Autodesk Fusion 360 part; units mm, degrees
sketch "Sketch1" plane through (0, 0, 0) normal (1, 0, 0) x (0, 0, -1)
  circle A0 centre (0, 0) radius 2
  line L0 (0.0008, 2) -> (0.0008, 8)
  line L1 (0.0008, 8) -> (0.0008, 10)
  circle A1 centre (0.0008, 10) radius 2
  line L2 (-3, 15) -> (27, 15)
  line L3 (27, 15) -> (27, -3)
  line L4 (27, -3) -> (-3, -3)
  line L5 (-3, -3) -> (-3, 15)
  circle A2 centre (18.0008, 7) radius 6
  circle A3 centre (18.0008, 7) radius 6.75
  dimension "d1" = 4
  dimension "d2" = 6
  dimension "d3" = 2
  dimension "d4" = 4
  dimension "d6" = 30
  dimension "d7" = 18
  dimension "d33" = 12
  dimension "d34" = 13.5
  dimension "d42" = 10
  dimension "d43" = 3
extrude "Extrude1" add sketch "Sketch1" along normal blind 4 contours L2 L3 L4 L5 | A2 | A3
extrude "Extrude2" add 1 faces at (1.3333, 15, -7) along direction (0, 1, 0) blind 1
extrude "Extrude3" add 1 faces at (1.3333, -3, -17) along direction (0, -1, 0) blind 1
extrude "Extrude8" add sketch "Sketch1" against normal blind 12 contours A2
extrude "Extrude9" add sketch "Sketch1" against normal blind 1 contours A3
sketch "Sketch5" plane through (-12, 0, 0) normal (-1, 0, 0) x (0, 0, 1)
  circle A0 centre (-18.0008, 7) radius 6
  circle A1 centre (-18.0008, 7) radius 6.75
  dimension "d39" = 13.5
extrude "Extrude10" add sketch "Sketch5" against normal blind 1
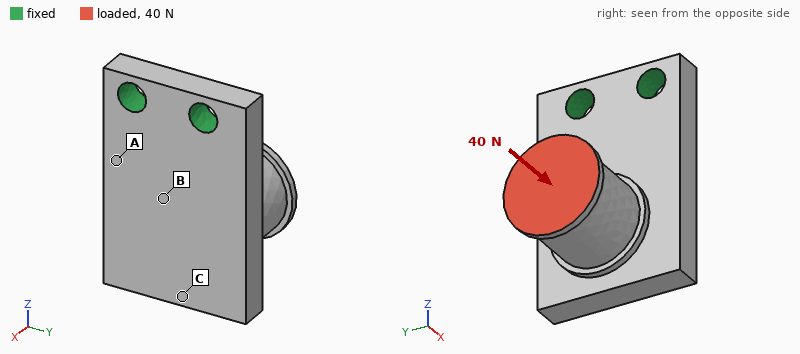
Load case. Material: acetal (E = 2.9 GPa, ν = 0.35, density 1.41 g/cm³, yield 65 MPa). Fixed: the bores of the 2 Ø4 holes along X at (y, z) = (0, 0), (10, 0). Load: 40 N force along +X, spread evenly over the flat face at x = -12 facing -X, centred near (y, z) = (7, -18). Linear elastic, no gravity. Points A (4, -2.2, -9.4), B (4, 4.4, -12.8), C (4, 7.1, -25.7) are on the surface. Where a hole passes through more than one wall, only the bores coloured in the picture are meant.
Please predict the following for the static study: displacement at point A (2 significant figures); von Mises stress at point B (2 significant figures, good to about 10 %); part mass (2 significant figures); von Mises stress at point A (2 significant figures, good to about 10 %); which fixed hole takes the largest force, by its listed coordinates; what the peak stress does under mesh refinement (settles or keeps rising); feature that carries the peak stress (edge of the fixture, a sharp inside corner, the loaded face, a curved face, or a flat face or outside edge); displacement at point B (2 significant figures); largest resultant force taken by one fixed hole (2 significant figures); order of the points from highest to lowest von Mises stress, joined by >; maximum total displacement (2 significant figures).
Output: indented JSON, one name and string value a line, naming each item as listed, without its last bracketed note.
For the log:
{
  "displacement at point A": "0.064 mm",
  "von Mises stress at point B": "3.6 MPa",
  "part mass": "5.2 g",
  "von Mises stress at point A": "6.4 MPa",
  "which fixed hole takes the largest force, by its listed coordinates": "(10, 0)",
  "what the peak stress does under mesh refinement": "keeps rising",
  "feature that carries the peak stress": "edge of the fixture",
  "displacement at point B": "0.12 mm",
  "largest resultant force taken by one fixed hole": "26 N",
  "order of the points from highest to lowest von Mises stress, joined by >": "A > B > C",
  "maximum total displacement": "0.41 mm"
}
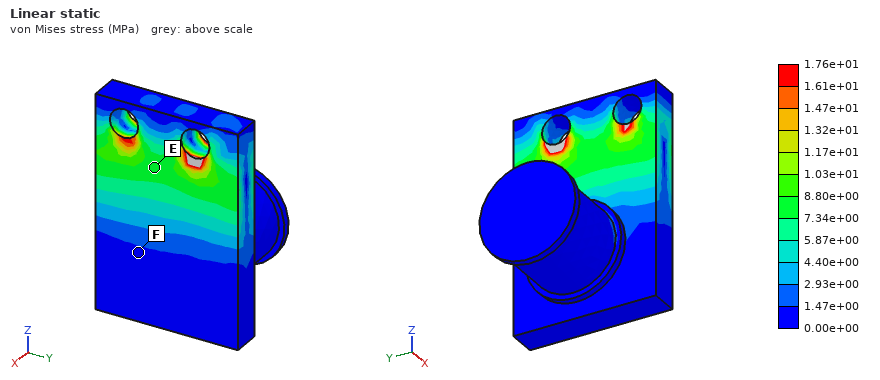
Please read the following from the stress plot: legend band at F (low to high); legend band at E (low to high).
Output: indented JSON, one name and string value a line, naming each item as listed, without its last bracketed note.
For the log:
{
  "legend band at F": "0.00e+00 to 1.47e+00 MPa",
  "legend band at E": "7.34e+00 to 8.80e+00 MPa"
}
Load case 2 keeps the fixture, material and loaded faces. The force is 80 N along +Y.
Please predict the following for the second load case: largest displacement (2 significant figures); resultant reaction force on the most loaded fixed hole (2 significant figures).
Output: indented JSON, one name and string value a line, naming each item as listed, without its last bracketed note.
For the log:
{
  "largest displacement": "0.42 mm",
  "resultant reaction force on the most loaded fixed hole": "140 N"
}
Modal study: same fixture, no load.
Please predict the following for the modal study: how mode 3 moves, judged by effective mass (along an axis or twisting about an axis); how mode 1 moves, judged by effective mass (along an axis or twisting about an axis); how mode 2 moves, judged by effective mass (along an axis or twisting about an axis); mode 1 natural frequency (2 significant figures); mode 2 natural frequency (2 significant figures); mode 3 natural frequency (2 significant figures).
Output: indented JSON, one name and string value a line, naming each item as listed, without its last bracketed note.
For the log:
{
  "how mode 3 moves, judged by effective mass": "along Y",
  "how mode 1 moves, judged by effective mass": "along X",
  "how mode 2 moves, judged by effective mass": "along Y",
  "mode 1 natural frequency": "920 Hz",
  "mode 2 natural frequency": "2200 Hz",
  "mode 3 natural frequency": "4000 Hz"
}
